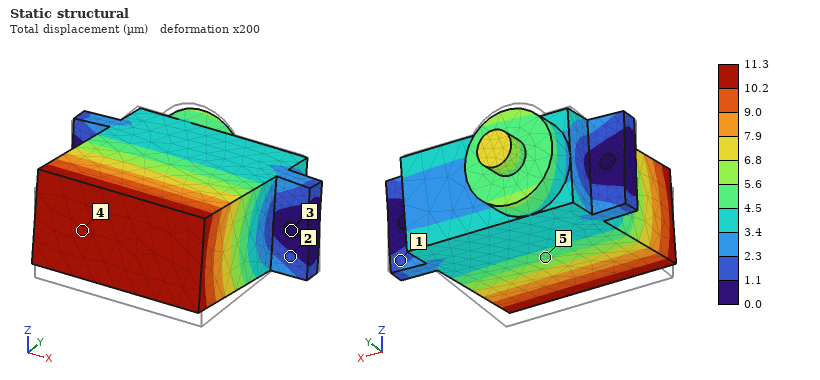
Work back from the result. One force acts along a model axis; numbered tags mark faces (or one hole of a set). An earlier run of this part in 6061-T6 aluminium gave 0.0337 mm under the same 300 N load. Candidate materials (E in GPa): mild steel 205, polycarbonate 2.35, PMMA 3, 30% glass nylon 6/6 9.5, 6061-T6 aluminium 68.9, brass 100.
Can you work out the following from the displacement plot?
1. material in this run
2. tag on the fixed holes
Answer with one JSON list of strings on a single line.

["mild steel", "3"]
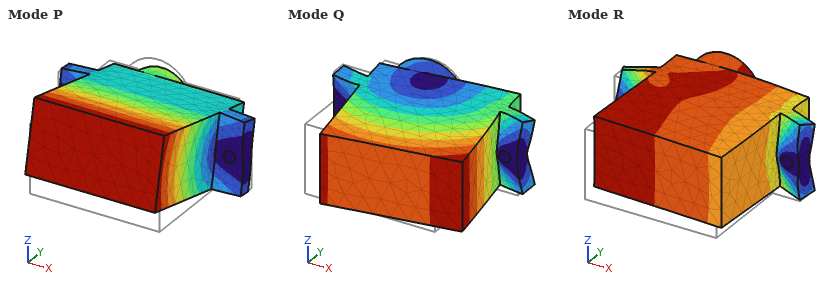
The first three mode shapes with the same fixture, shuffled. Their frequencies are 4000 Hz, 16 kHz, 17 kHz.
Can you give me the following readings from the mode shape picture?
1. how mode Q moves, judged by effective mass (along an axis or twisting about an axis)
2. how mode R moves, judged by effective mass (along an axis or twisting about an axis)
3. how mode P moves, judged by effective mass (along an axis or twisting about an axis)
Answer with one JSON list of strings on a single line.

["along X", "along Y", "along Z"]
